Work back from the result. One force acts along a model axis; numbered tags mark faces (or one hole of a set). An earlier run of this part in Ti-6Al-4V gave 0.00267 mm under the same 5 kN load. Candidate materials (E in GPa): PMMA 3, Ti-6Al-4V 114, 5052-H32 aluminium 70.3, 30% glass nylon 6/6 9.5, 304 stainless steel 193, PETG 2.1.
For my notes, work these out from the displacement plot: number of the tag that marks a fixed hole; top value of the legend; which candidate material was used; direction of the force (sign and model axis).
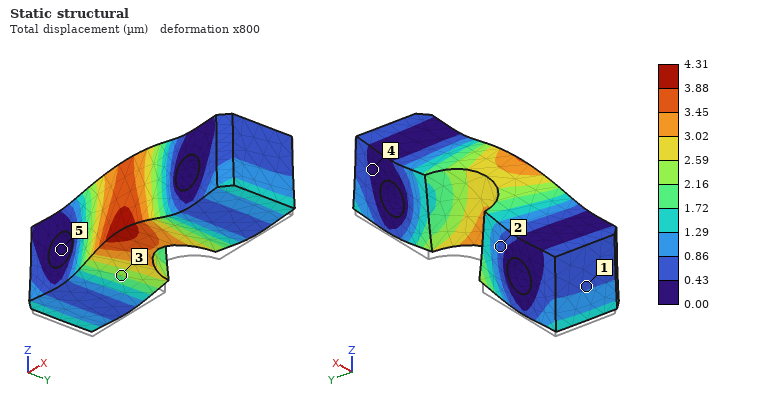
5
4.31 µm
5052-H32 aluminium
+Z
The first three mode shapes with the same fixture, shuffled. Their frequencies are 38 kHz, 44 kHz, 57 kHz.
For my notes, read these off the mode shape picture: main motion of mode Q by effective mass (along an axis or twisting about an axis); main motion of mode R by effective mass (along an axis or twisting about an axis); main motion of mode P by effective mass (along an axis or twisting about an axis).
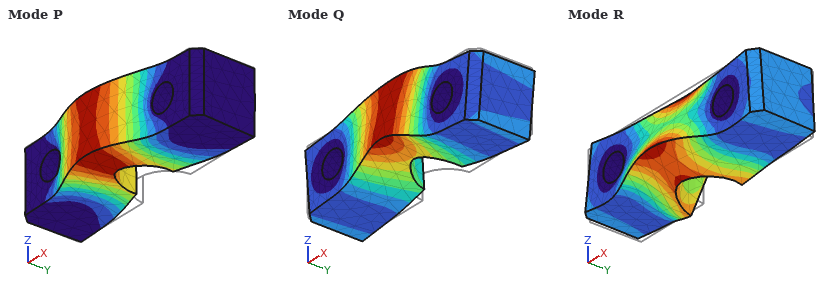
along Z
twisting about X
along Y
